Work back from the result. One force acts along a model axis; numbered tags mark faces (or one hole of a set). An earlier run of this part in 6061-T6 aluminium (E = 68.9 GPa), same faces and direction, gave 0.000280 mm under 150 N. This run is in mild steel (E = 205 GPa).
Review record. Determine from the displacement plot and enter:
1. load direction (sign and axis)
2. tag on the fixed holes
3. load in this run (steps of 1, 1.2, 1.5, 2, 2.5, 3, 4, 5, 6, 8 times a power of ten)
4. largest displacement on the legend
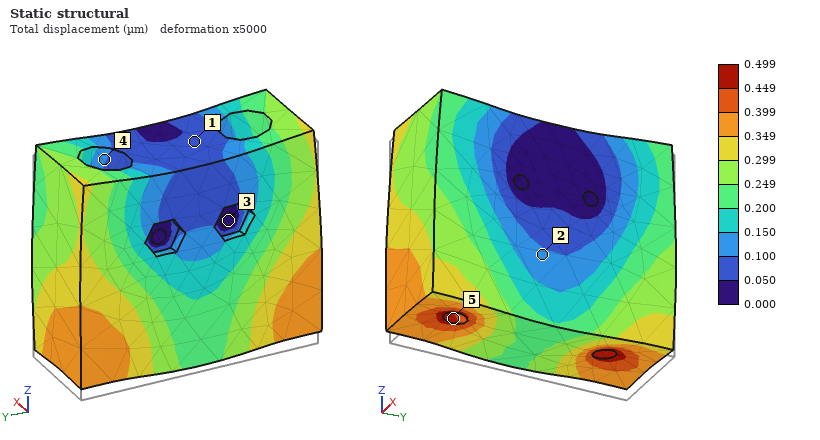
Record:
+Z
3
800 N
0.499 µm
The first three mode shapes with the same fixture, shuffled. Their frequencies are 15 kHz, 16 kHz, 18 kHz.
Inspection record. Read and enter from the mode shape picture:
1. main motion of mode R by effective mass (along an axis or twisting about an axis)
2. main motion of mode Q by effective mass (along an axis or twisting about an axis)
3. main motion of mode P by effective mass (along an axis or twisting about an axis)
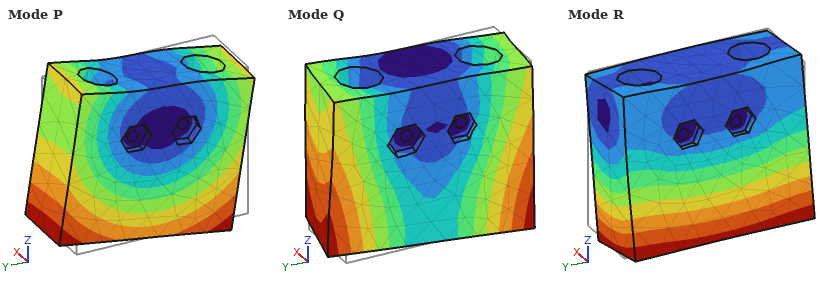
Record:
along X
twisting about Z
along Y
